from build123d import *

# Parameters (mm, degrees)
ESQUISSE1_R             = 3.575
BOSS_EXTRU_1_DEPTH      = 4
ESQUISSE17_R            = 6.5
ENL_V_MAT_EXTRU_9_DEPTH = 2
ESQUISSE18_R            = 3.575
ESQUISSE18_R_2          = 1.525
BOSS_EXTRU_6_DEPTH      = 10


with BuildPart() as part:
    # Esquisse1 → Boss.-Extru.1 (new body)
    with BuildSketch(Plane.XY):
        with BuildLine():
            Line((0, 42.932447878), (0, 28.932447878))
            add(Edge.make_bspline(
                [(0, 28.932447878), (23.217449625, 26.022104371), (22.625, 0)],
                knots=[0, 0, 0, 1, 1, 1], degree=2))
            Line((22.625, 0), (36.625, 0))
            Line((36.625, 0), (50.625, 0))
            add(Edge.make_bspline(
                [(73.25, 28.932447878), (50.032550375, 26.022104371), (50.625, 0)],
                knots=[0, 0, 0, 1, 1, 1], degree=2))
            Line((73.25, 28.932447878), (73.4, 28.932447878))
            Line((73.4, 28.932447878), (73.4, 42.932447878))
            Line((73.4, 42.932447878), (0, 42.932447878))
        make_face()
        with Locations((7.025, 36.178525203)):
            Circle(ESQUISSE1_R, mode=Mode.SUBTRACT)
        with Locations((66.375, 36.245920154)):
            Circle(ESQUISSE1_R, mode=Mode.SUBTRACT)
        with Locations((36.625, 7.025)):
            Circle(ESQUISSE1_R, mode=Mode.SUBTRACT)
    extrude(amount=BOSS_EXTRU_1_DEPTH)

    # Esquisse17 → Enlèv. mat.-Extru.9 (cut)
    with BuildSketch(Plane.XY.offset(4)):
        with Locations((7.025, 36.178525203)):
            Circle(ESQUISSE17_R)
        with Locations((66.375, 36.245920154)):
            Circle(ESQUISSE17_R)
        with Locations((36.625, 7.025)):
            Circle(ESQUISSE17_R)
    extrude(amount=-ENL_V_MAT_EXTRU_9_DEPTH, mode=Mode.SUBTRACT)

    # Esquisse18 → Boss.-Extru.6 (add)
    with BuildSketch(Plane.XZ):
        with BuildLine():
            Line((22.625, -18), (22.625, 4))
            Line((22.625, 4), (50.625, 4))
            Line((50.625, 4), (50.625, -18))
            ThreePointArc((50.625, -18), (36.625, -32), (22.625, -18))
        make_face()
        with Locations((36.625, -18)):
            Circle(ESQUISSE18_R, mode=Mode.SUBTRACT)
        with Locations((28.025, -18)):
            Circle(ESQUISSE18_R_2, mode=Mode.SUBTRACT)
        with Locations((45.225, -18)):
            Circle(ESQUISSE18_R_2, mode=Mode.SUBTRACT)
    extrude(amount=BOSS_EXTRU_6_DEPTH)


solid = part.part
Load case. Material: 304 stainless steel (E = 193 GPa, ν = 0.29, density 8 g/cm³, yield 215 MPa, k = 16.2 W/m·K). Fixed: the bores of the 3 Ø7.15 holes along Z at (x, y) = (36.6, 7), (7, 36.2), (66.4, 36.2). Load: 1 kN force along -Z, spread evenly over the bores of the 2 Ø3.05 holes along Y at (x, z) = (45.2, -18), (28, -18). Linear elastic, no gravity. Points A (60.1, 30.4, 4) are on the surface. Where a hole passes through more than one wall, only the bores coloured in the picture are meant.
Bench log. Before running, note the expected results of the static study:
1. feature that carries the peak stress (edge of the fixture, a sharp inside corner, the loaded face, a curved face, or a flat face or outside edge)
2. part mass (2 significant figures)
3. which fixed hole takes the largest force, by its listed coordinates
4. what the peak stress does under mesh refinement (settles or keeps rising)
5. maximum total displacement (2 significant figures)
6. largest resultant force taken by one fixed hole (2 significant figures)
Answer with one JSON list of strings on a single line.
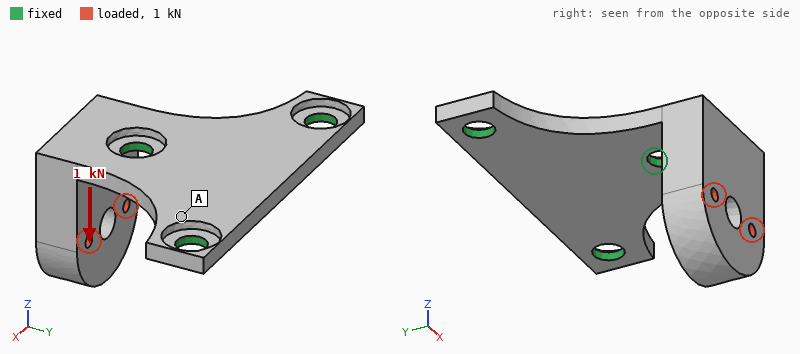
["edge of the fixture", "130 g", "(36.6, 7)", "keeps rising", "0.13 mm", "1.2 kN"]
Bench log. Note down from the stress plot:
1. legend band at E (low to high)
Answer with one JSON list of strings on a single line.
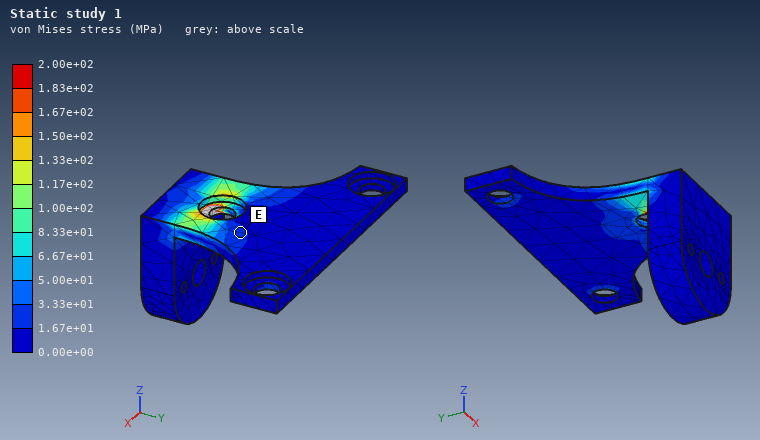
["1.67e+01 to 3.33e+01 MPa"]
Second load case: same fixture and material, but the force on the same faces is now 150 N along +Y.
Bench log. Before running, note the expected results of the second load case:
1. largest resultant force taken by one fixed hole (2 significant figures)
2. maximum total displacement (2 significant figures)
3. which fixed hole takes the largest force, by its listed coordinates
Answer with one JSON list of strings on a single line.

["270 N", "48 µm", "(36.6, 7)"]
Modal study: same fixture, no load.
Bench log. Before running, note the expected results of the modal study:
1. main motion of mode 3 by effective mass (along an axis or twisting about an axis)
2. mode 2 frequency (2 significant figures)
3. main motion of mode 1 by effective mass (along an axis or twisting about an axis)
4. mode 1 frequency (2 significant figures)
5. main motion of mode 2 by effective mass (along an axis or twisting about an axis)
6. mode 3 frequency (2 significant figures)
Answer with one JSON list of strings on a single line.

["along Z", "2300 Hz", "along Y", "1500 Hz", "along X", "6100 Hz"]
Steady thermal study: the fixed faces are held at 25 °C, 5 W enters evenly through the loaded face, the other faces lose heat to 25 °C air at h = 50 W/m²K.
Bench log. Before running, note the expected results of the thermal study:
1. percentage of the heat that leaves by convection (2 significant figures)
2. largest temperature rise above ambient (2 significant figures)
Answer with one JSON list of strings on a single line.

["68 %", "28 K"]
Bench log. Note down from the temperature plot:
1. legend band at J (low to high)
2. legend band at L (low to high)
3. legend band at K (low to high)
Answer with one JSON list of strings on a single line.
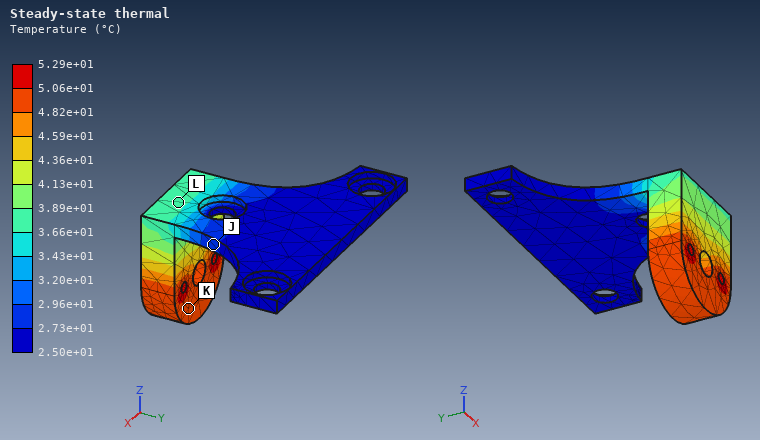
["2.73e+01 to 2.96e+01 °C", "3.66e+01 to 3.89e+01 °C", "4.82e+01 to 5.06e+01 °C"]
